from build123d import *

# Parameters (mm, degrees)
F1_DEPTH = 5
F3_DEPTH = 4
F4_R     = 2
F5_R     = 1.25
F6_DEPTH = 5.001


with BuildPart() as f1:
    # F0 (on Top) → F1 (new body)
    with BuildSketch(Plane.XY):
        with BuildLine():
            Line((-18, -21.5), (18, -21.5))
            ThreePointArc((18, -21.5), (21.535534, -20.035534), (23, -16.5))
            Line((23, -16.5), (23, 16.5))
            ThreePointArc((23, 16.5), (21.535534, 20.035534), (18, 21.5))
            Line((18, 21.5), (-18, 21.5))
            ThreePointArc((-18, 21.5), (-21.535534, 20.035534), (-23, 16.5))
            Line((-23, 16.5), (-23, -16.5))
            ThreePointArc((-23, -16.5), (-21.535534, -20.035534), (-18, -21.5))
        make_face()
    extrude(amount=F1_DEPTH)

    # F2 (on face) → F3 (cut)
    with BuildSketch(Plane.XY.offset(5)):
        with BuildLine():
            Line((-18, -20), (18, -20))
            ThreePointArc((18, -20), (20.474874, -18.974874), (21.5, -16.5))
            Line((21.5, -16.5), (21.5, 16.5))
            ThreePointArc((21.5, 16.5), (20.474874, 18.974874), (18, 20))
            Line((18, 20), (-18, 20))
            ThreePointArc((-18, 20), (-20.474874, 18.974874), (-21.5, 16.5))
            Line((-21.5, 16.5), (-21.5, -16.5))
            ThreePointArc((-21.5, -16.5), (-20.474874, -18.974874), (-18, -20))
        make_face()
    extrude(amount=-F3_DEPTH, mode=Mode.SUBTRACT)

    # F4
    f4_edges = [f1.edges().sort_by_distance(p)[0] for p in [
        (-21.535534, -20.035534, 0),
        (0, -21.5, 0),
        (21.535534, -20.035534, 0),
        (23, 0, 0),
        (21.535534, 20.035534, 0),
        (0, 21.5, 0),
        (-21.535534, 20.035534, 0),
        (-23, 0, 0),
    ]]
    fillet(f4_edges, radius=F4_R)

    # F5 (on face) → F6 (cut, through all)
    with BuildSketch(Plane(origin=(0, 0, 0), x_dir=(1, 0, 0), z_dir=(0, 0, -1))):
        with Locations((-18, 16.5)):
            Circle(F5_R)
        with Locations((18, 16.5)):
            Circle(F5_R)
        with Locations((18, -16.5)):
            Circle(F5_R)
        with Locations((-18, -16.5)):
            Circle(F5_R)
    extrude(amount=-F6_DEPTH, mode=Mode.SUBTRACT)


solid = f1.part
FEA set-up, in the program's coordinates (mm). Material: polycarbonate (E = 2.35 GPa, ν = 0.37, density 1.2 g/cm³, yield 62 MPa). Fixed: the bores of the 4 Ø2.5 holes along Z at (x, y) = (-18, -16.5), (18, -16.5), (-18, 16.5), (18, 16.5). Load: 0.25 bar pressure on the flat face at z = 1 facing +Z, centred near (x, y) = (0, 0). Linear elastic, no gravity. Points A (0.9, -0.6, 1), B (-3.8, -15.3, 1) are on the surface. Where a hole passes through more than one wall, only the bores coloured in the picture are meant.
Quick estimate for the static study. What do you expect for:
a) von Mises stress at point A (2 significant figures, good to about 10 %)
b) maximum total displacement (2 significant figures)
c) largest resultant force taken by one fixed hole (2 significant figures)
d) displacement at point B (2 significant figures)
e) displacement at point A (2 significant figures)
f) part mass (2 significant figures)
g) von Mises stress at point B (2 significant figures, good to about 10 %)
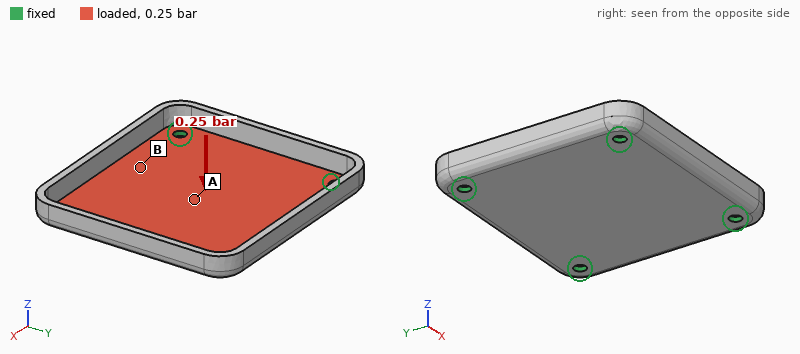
8.1 MPa
0.71 mm
12 N
0.26 mm
0.71 mm
3.3 g
3.1 MPa
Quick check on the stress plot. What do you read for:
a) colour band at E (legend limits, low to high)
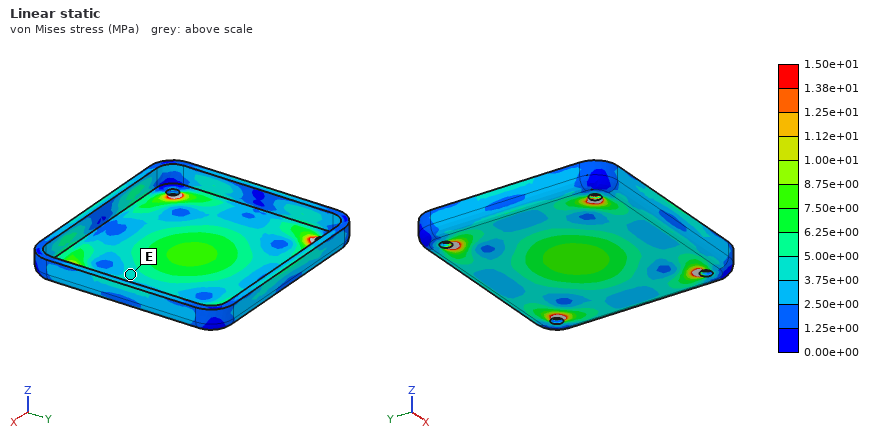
3.75e+00 to 5.00e+00 MPa
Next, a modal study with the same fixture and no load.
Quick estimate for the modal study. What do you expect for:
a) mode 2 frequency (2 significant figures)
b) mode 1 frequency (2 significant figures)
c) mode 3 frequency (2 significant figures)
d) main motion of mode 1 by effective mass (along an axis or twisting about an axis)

2200 Hz
1100 Hz
2200 Hz
along Z
